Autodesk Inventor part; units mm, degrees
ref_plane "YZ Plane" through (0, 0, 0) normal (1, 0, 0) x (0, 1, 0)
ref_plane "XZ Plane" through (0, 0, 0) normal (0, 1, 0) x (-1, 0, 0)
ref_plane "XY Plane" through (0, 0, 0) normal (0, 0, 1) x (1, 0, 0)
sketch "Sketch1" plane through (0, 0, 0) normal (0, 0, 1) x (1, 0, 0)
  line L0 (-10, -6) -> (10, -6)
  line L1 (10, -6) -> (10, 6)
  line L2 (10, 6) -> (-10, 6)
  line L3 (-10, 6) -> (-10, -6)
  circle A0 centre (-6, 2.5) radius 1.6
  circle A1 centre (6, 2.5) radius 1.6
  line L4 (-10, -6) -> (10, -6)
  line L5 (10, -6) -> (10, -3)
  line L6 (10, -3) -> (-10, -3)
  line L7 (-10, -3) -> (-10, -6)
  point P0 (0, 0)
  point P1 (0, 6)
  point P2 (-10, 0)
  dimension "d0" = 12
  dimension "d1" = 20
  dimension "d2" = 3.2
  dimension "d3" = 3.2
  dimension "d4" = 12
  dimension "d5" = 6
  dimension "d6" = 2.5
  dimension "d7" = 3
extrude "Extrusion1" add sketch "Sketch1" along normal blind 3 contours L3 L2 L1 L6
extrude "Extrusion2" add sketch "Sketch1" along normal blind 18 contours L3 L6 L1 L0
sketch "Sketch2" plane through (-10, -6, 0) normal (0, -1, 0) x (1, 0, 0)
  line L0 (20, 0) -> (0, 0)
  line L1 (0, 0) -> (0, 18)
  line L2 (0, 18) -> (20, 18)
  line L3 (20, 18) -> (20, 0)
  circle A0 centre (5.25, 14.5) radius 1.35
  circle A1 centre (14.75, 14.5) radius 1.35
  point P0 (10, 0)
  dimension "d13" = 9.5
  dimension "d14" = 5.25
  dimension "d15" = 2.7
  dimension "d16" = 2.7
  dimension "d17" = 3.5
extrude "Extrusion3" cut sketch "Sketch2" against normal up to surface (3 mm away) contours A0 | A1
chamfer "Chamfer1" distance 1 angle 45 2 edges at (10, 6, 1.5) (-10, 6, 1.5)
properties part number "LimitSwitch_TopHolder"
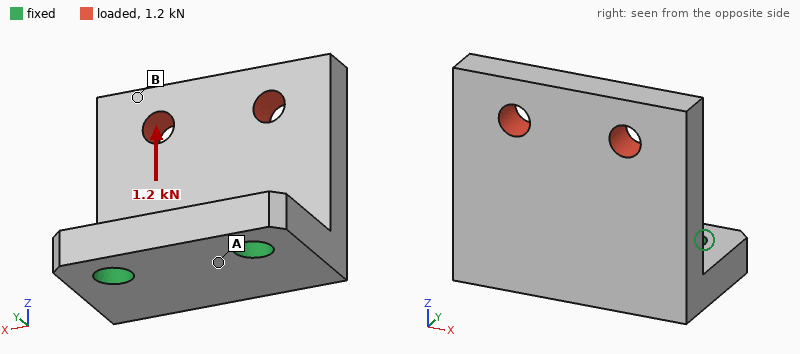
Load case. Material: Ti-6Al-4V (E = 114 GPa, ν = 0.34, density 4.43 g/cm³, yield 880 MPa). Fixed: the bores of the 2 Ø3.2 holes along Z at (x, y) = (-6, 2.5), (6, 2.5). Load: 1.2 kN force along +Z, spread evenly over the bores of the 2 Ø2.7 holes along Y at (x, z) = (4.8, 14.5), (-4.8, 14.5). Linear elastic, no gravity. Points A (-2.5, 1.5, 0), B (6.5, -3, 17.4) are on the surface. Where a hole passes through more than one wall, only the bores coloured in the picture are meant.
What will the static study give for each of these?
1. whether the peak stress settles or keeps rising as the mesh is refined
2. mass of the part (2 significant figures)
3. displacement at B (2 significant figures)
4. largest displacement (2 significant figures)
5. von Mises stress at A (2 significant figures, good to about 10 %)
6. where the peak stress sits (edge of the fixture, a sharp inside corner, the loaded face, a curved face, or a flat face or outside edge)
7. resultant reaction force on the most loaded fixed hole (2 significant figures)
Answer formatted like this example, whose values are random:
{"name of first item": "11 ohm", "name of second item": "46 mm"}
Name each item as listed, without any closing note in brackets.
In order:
{"whether the peak stress settles or keeps rising as the mesh is refined": "keeps rising", "mass of the part": "6.8 g", "displacement at B": "79 µm", "largest displacement": "86 µm", "von Mises stress at A": "99 MPa", "where the peak stress sits": "edge of the fixture", "resultant reaction force on the most loaded fixed hole": "600 N"}
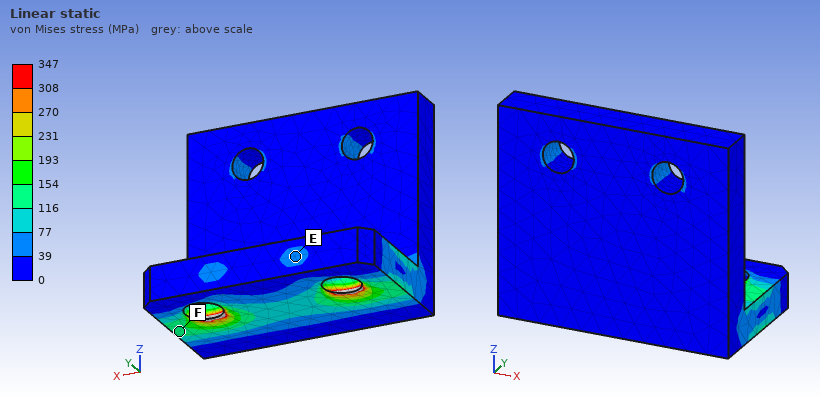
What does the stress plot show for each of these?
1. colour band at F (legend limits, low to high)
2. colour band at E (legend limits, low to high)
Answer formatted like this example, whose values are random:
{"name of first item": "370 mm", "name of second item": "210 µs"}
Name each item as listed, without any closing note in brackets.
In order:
{"colour band at F": "116 to 154 MPa", "colour band at E": "39 to 77 MPa"}
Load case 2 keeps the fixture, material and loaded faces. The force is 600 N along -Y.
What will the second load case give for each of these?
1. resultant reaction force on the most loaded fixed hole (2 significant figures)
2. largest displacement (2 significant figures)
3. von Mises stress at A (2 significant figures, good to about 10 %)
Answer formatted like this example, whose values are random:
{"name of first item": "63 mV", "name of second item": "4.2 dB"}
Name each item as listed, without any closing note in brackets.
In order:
{"resultant reaction force on the most loaded fixed hole": "330 N", "largest displacement": "0.25 mm", "von Mises stress at A": "120 MPa"}
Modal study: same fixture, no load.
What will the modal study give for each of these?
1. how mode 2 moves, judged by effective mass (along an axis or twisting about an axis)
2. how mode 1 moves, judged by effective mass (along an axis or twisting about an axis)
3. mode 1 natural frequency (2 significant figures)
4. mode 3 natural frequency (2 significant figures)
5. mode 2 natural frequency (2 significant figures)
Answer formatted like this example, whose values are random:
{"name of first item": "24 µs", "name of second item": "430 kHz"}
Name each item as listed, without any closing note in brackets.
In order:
{"how mode 2 moves, judged by effective mass": "along X", "how mode 1 moves, judged by effective mass": "along Y", "mode 1 natural frequency": "6000 Hz", "mode 3 natural frequency": "18 kHz", "mode 2 natural frequency": "12 kHz"}
